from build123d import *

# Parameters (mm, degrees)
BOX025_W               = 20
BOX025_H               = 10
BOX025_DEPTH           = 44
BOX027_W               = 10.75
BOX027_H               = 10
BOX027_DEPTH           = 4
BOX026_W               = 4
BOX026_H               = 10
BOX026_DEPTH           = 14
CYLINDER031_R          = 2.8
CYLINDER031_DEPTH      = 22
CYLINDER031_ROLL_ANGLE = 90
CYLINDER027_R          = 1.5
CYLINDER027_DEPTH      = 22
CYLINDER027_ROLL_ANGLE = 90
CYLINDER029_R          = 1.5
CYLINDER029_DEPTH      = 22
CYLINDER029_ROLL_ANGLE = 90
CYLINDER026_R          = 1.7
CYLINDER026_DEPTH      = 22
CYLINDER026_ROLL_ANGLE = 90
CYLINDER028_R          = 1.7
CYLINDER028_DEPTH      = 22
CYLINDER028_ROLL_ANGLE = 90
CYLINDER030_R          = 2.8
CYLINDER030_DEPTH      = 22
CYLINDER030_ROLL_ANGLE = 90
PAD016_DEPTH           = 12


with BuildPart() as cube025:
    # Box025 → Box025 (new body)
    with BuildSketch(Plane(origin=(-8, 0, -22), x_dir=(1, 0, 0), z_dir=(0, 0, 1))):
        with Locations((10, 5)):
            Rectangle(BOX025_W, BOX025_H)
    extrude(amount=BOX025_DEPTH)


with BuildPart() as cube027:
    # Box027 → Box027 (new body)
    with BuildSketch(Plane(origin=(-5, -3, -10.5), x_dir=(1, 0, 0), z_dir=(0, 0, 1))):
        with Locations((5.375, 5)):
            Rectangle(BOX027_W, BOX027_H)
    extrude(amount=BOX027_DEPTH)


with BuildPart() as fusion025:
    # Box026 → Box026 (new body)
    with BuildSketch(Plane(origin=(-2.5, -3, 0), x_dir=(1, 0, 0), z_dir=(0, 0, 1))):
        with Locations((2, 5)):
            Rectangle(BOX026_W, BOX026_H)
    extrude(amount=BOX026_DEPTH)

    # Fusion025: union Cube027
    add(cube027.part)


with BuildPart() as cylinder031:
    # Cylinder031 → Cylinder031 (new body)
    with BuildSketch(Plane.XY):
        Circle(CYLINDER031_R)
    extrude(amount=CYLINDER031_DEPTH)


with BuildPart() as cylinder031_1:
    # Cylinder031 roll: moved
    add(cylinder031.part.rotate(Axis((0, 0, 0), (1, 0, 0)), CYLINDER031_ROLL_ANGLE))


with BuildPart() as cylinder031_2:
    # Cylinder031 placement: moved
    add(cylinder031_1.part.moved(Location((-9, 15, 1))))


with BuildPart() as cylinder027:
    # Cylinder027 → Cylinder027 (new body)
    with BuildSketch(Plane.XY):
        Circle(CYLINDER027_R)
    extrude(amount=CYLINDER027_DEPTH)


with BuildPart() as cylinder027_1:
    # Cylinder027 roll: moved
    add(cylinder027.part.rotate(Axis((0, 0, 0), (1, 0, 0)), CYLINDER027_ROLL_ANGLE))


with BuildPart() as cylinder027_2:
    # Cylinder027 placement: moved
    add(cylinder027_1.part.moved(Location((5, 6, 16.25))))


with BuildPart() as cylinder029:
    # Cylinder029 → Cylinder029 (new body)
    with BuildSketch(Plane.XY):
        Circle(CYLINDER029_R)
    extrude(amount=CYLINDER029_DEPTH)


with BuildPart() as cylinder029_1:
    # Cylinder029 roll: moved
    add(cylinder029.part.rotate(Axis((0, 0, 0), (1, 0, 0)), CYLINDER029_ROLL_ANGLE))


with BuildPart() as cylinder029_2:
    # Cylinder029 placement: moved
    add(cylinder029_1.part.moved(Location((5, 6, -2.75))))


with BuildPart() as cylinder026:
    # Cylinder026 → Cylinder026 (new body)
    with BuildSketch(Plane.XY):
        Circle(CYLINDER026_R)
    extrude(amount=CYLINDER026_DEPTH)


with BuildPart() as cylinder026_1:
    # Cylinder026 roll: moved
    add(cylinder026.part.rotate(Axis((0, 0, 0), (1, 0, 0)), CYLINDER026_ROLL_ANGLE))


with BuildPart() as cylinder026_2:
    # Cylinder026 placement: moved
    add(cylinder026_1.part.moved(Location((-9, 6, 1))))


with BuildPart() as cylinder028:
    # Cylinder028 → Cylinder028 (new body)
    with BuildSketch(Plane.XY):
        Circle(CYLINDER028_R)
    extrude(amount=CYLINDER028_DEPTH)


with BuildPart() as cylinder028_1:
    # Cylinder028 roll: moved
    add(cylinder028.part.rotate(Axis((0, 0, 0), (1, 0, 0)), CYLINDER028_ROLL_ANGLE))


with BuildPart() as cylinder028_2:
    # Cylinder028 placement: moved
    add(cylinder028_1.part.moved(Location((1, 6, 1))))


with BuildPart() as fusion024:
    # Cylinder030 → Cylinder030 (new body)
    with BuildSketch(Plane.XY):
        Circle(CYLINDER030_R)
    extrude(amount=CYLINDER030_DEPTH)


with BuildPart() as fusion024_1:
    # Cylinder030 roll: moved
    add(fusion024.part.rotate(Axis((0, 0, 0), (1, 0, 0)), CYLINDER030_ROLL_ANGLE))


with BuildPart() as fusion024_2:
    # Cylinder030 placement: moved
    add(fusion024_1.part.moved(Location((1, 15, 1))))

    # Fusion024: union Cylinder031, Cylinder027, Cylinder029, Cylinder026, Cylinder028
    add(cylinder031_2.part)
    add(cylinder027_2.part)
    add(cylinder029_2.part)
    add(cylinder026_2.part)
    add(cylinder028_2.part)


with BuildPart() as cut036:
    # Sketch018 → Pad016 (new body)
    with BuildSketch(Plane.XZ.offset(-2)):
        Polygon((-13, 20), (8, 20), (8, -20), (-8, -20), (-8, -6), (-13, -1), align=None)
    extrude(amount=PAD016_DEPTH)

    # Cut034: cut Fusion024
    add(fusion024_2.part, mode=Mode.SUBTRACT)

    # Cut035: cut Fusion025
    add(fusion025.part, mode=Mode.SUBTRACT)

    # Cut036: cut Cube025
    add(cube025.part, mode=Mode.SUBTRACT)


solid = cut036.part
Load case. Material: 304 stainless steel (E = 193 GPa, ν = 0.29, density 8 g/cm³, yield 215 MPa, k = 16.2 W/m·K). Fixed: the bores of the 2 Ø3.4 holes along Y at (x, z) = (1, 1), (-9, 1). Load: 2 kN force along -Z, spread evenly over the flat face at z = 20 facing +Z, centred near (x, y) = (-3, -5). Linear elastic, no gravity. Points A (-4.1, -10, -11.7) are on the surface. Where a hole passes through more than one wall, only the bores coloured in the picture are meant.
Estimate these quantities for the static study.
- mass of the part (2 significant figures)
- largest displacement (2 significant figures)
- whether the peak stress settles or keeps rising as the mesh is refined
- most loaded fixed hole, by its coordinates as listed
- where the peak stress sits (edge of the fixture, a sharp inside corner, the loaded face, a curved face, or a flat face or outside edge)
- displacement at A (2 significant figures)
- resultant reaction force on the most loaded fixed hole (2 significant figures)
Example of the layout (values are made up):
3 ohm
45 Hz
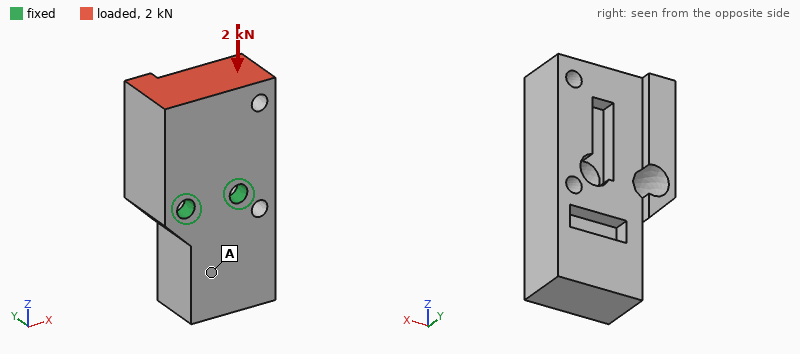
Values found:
56 g
17 µm
keeps rising
(1, 1)
edge of the fixture
8.4 µm
1.2 kN
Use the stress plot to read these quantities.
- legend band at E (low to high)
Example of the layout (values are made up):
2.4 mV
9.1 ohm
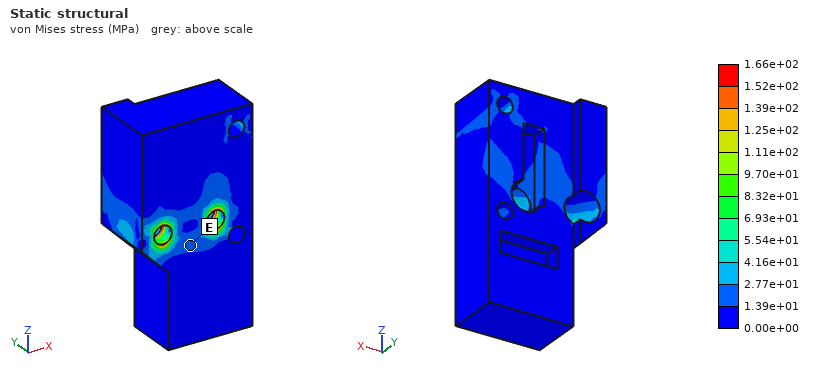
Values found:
1.39e+01 to 2.77e+01 MPa
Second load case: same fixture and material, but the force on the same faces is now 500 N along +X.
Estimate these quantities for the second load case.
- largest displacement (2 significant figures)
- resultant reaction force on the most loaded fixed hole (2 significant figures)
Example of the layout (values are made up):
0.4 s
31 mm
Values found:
4.0 µm
830 N
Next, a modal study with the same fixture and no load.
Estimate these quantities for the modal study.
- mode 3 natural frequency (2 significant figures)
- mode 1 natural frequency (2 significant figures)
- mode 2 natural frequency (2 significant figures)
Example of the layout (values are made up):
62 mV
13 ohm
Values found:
14 kHz
5500 Hz
14 kHz
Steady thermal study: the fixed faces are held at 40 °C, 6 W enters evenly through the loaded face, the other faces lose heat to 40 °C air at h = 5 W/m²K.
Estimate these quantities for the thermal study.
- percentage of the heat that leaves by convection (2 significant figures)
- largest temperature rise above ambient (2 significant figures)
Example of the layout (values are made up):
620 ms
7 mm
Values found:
4.2 %
45 K
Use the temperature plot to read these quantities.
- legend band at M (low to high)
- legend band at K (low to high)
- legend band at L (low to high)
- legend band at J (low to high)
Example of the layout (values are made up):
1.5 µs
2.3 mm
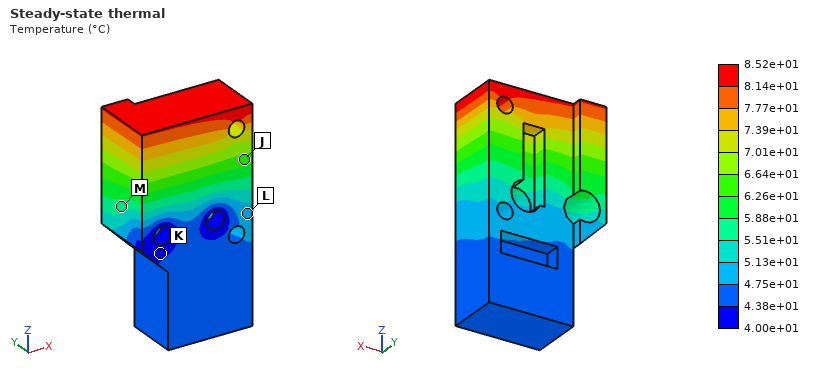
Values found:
5.51e+01 to 5.88e+01 °C
4.00e+01 to 4.38e+01 °C
4.75e+01 to 5.13e+01 °C
6.26e+01 to 6.64e+01 °C
